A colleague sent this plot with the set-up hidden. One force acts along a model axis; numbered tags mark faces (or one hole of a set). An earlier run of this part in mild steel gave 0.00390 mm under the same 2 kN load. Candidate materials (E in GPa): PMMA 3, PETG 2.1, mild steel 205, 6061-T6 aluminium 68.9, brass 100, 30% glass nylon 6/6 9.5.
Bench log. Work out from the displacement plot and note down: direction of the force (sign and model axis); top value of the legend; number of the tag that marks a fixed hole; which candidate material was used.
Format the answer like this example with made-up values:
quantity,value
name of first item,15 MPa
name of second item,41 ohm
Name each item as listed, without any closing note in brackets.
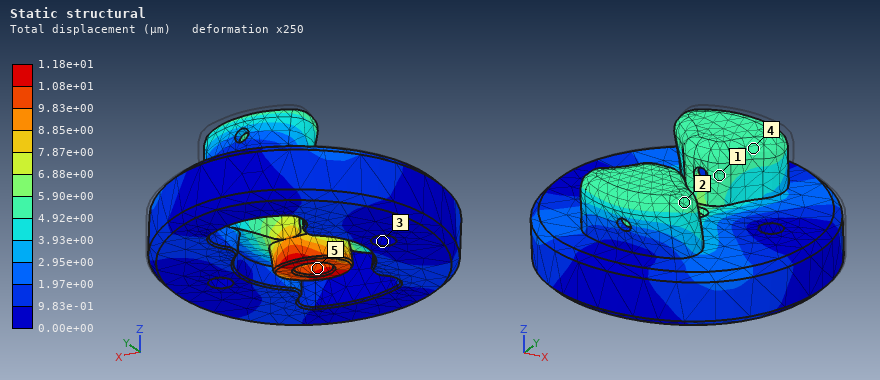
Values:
quantity,value
direction of the force,-Y
top value of the legend,1.18e+01 µm
number of the tag that marks a fixed hole,3
which candidate material was used,6061-T6 aluminium
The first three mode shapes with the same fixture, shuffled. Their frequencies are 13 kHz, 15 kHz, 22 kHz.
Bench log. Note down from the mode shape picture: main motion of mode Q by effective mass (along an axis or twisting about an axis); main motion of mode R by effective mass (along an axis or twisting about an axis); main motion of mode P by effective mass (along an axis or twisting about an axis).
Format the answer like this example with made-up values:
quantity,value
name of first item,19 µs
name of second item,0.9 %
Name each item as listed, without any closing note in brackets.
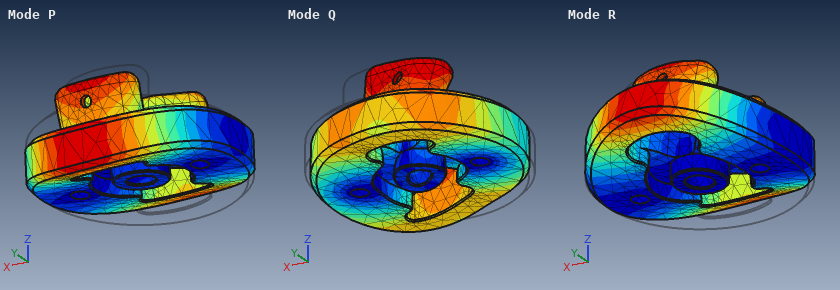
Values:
quantity,value
main motion of mode Q by effective mass,twisting about Z
main motion of mode R by effective mass,along Z
main motion of mode P by effective mass,twisting about X
